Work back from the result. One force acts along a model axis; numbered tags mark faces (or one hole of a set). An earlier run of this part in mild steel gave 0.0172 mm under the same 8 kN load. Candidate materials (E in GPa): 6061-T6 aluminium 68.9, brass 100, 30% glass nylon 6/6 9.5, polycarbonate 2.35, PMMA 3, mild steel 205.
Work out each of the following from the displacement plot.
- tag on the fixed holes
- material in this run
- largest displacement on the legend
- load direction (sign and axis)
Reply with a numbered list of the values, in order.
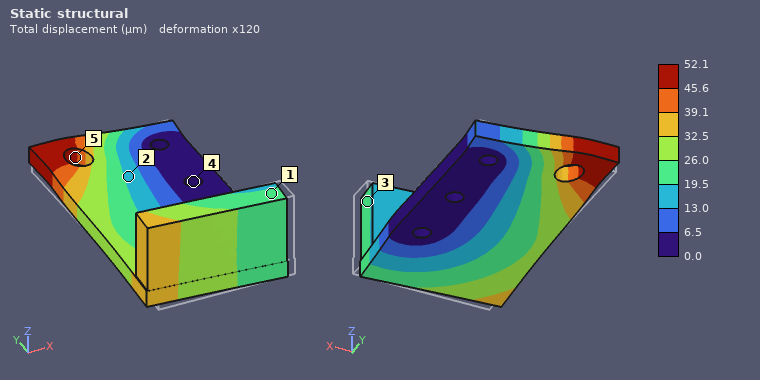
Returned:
1. 4
2. 6061-T6 aluminium
3. 52.1 µm
4. +Y
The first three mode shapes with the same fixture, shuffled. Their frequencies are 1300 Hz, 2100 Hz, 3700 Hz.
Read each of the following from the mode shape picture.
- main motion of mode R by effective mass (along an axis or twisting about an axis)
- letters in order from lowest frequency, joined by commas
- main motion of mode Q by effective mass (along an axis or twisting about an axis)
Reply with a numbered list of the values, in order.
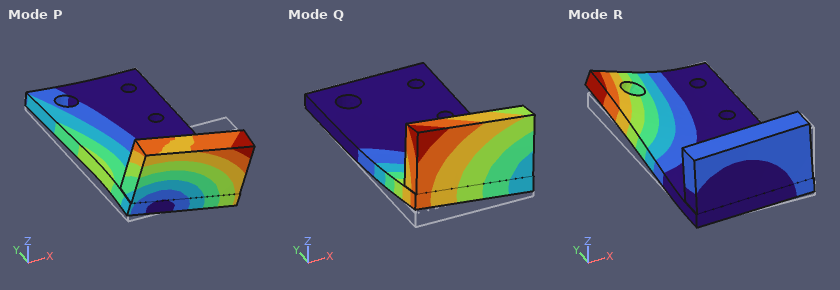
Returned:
1. along Z
2. Q, P, R
3. along Z
